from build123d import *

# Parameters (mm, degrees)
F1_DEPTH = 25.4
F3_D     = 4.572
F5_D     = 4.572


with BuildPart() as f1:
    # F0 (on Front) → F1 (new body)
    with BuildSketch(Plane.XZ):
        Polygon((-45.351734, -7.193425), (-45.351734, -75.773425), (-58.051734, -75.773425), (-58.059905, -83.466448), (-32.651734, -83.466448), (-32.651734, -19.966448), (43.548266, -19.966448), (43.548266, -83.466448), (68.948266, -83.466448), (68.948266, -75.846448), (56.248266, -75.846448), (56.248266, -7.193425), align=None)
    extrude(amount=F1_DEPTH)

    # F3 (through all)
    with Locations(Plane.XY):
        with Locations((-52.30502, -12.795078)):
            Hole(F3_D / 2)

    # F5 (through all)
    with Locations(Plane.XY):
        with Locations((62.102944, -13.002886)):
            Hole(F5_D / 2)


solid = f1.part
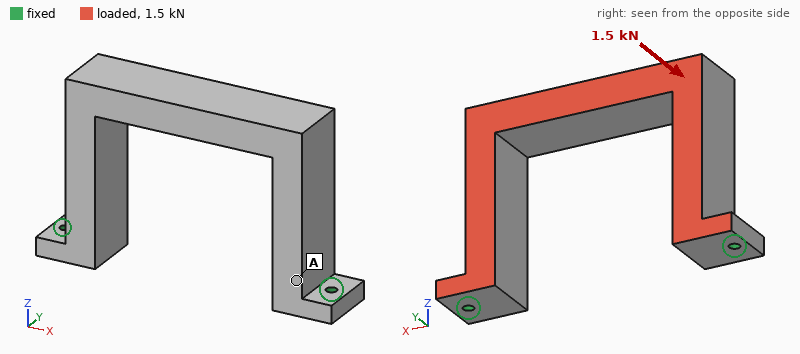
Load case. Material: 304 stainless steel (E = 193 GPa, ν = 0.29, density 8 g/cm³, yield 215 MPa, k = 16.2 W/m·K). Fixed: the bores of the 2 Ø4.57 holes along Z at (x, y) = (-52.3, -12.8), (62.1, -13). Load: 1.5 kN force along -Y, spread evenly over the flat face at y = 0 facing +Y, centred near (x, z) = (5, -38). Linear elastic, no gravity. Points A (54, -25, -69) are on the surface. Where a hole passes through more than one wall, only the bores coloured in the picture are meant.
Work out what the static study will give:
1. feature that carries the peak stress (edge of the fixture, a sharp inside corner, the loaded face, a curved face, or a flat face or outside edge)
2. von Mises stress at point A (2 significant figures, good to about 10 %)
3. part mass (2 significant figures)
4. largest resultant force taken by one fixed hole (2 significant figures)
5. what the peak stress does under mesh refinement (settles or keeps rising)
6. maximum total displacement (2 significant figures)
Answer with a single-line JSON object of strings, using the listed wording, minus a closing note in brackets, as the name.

{"feature that carries the peak stress": "edge of the fixture", "von Mises stress at point A": "26 MPa", "part mass": "630 g", "largest resultant force taken by one fixed hole": "760 N", "what the peak stress does under mesh refinement": "keeps rising", "maximum total displacement": "0.11 mm"}
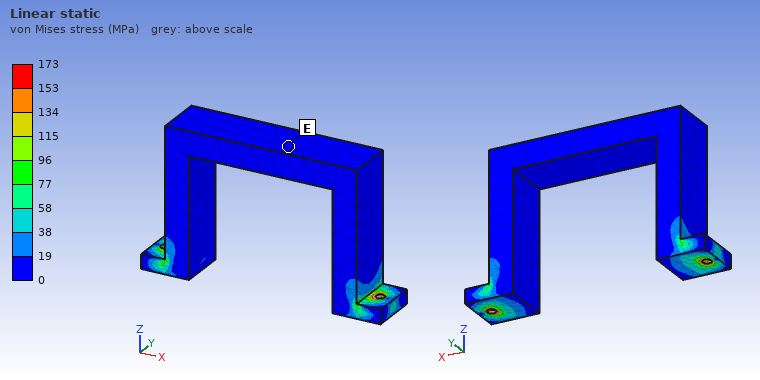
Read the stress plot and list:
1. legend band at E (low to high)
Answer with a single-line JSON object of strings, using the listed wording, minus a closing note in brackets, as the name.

{"legend band at E": "0 to 19 MPa"}
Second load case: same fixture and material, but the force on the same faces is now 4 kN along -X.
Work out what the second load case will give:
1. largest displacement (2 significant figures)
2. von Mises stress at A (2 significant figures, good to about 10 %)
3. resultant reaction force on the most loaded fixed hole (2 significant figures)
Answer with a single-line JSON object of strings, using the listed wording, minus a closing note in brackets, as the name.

{"largest displacement": "0.12 mm", "von Mises stress at A": "24 MPa", "resultant reaction force on the most loaded fixed hole": "2.3 kN"}
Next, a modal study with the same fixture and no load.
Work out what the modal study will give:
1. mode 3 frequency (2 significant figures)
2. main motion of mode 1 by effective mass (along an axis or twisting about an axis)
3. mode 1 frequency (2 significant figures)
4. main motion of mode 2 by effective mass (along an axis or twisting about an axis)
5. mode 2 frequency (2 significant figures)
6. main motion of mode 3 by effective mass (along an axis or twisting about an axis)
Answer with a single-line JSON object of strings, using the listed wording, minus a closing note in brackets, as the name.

{"mode 3 frequency": "1900 Hz", "main motion of mode 1 by effective mass": "along Y", "mode 1 frequency": "830 Hz", "main motion of mode 2 by effective mass": "along X", "mode 2 frequency": "1300 Hz", "main motion of mode 3 by effective mass": "twisting about Z"}
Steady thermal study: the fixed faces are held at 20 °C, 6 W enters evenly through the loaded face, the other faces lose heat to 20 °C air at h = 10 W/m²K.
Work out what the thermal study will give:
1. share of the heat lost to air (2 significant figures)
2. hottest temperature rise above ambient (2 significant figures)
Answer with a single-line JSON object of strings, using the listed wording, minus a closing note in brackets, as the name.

{"share of the heat lost to air": "39 %", "hottest temperature rise above ambient": "22 K"}
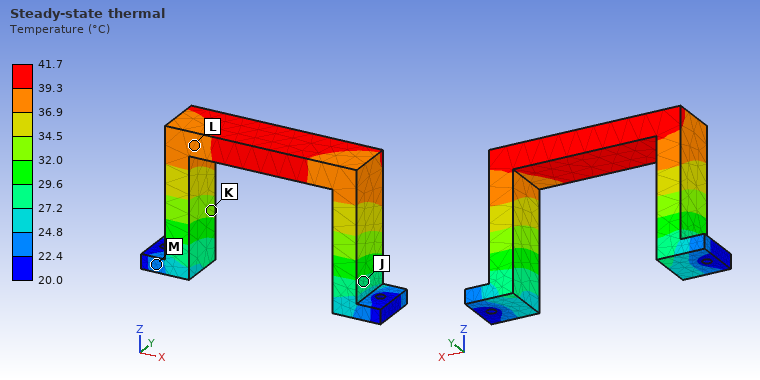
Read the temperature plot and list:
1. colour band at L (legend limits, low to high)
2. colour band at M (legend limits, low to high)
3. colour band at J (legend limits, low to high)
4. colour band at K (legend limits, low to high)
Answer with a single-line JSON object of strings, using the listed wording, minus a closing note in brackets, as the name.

{"colour band at L": "36.9 to 39.3 °C", "colour band at M": "22.4 to 24.8 °C", "colour band at J": "27.2 to 29.6 °C", "colour band at K": "32.0 to 34.5 °C"}
